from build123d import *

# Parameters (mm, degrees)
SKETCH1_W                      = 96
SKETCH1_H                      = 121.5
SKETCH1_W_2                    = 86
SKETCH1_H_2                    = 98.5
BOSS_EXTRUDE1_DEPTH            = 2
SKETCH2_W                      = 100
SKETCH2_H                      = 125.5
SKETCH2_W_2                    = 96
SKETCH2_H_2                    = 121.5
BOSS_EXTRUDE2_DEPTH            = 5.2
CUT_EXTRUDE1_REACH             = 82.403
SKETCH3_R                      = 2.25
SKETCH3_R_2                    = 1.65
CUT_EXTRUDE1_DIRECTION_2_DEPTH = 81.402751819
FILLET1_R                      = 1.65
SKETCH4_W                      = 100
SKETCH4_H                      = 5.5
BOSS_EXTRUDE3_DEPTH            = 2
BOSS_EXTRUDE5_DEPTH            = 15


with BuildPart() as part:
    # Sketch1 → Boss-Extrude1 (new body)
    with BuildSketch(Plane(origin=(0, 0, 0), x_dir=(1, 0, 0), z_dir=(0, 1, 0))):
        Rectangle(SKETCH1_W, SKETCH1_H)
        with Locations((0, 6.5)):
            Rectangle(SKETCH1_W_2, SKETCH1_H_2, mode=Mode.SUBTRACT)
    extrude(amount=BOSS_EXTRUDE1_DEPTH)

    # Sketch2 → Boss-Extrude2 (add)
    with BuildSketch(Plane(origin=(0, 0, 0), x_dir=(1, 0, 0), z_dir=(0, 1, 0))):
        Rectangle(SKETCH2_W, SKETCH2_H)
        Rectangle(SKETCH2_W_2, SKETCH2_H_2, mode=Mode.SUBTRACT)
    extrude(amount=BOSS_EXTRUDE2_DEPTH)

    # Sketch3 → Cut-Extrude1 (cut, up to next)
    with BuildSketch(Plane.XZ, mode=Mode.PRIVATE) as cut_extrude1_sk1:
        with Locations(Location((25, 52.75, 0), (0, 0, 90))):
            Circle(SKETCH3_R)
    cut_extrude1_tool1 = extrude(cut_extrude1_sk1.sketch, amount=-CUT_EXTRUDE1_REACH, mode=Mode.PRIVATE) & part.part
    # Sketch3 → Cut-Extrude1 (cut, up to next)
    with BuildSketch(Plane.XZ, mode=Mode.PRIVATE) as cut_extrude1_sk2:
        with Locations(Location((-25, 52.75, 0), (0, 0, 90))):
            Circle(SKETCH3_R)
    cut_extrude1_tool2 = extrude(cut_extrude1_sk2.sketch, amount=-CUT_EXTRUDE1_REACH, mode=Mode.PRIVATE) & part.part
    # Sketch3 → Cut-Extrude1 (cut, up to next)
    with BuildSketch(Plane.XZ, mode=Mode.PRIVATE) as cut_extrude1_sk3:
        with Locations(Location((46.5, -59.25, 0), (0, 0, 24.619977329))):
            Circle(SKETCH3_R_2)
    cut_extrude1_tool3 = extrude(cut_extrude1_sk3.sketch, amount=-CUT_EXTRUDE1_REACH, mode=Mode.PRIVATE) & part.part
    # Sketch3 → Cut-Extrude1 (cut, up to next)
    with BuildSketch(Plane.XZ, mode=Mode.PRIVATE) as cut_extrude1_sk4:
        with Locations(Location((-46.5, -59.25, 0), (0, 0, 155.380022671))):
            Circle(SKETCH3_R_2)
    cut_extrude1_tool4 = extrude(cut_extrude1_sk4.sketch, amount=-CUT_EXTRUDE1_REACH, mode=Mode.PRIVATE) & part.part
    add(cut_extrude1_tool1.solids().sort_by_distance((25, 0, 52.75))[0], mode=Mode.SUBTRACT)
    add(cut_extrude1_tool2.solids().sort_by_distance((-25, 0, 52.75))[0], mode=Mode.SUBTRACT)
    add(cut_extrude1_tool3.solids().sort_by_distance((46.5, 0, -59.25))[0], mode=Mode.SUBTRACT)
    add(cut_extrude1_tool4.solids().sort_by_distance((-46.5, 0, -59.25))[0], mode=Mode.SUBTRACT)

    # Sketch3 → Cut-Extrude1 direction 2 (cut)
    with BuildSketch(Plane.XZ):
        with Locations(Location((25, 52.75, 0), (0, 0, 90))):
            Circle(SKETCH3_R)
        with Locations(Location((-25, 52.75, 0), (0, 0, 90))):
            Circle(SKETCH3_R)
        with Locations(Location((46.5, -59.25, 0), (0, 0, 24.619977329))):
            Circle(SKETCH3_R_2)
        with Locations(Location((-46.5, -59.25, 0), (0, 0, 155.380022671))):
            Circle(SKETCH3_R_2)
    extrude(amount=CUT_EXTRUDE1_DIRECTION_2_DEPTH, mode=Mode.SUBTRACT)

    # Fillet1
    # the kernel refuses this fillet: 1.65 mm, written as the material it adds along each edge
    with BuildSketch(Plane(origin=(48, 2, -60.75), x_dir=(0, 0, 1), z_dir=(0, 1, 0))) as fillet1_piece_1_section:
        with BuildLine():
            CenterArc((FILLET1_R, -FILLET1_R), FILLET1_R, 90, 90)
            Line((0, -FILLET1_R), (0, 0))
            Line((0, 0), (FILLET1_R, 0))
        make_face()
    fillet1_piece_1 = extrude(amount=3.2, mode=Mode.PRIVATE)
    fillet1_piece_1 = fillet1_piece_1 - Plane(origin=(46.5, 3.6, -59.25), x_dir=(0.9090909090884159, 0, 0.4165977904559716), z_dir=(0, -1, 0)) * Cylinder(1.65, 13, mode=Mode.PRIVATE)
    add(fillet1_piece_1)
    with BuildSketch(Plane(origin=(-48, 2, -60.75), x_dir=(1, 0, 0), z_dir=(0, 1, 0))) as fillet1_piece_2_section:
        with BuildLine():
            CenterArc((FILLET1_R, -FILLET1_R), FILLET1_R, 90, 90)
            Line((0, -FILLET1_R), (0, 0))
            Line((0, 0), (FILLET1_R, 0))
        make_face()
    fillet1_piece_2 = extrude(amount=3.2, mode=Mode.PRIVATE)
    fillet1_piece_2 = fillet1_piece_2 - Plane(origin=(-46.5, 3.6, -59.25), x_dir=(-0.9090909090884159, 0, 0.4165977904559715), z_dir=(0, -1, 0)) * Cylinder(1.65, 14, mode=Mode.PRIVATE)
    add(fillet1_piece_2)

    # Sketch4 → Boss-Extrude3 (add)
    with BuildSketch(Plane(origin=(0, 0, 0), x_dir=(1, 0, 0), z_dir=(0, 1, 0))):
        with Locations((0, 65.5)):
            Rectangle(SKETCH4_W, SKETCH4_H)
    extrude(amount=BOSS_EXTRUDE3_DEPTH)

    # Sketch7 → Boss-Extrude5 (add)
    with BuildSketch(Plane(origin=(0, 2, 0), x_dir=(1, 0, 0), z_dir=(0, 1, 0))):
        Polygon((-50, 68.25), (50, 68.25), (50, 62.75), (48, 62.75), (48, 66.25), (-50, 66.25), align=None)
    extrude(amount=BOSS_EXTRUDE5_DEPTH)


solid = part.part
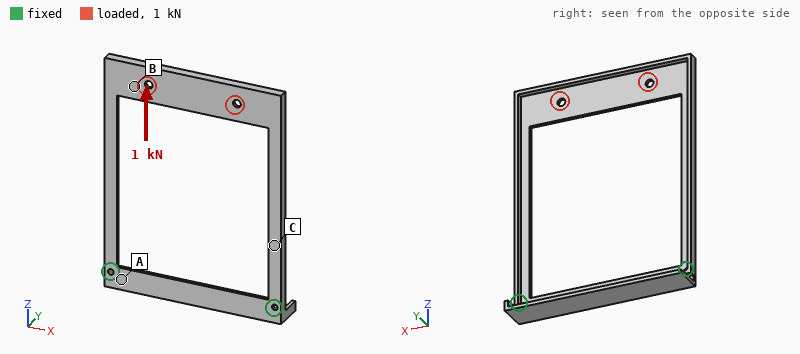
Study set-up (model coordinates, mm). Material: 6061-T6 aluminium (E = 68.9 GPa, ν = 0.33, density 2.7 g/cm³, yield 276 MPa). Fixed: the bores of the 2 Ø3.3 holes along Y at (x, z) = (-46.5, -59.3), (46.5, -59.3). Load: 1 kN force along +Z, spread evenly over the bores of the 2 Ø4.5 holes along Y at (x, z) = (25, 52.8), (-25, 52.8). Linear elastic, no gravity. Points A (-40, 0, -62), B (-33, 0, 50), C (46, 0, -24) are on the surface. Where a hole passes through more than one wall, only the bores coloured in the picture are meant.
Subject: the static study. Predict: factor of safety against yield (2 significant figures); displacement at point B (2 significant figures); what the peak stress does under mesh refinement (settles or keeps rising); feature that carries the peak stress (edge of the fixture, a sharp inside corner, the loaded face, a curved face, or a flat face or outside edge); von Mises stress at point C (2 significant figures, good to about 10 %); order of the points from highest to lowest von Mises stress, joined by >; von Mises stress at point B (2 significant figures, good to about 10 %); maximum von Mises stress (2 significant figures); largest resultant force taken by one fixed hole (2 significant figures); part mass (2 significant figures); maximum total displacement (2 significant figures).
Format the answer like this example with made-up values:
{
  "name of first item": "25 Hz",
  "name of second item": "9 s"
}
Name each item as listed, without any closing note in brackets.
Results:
{
  "factor of safety against yield": "3.0",
  "displacement at point B": "0.78 mm",
  "what the peak stress does under mesh refinement": "settles",
  "feature that carries the peak stress": "a flat face or outside edge",
  "von Mises stress at point C": "44 MPa",
  "order of the points from highest to lowest von Mises stress, joined by >": "C > B > A",
  "von Mises stress at point B": "28 MPa",
  "maximum von Mises stress": "92 MPa",
  "largest resultant force taken by one fixed hole": "500 N",
  "part mass": "41 g",
  "maximum total displacement": "1.1 mm"
}
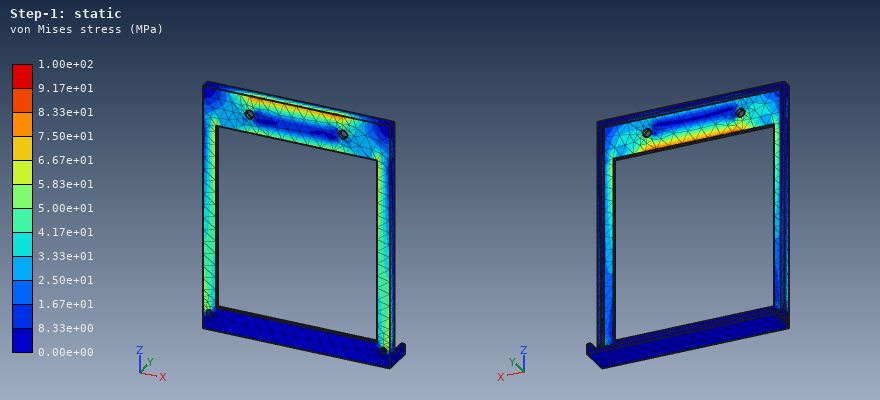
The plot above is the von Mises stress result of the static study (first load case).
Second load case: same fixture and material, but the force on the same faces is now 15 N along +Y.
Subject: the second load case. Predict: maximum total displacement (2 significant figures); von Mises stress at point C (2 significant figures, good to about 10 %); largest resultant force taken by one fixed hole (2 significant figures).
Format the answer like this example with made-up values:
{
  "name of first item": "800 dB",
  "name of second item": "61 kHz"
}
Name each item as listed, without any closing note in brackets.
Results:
{
  "maximum total displacement": "1.5 mm",
  "von Mises stress at point C": "26 MPa",
  "largest resultant force taken by one fixed hole": "18 N"
}
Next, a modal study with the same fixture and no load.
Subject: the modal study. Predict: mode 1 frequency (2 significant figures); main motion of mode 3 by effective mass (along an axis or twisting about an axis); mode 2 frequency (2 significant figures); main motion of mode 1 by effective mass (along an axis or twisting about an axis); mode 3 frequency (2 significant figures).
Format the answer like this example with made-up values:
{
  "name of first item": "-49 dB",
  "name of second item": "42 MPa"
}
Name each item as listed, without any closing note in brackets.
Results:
{
  "mode 1 frequency": "140 Hz",
  "main motion of mode 3 by effective mass": "along X",
  "mode 2 frequency": "260 Hz",
  "main motion of mode 1 by effective mass": "along Y",
  "mode 3 frequency": "420 Hz"
}
